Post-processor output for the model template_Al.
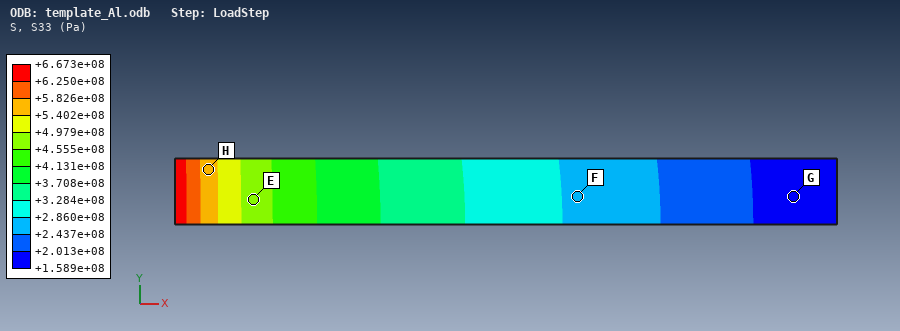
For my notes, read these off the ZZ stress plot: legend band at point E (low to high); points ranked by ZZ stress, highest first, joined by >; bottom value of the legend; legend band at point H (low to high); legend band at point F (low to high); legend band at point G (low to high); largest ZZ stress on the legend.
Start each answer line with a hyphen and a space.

- +4.555e+08 to +4.979e+08 Pa
- H > E > F > G
- +1.589e+08 Pa
- +5.402e+08 to +5.826e+08 Pa
- +2.437e+08 to +2.860e+08 Pa
- +1.589e+08 to +2.013e+08 Pa
- +6.673e+08 Pa
